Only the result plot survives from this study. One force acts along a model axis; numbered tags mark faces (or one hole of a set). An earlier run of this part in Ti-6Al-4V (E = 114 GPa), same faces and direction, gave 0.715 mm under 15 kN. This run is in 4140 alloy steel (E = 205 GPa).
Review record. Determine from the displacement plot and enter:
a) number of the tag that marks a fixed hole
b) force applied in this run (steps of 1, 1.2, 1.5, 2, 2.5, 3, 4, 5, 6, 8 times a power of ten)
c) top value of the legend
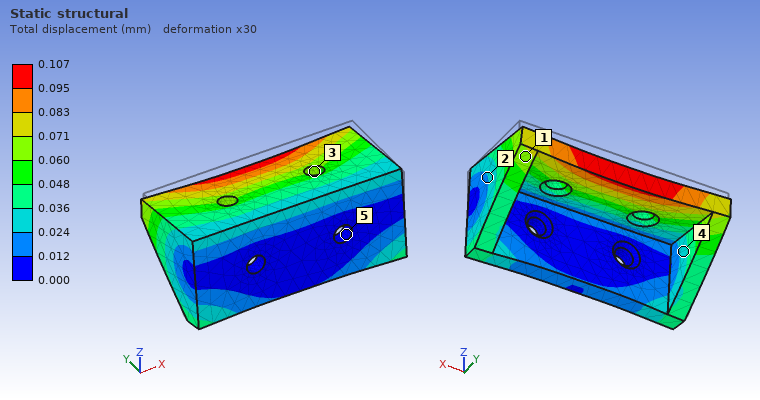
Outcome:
5
4 kN
0.107 mm
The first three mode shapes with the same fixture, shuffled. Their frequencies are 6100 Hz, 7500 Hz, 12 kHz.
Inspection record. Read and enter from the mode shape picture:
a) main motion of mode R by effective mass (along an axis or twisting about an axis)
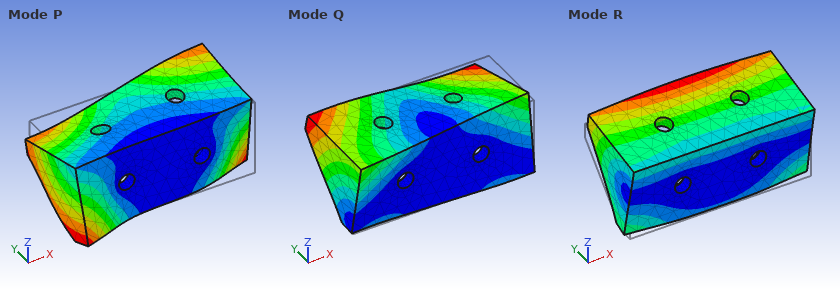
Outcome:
along Z
